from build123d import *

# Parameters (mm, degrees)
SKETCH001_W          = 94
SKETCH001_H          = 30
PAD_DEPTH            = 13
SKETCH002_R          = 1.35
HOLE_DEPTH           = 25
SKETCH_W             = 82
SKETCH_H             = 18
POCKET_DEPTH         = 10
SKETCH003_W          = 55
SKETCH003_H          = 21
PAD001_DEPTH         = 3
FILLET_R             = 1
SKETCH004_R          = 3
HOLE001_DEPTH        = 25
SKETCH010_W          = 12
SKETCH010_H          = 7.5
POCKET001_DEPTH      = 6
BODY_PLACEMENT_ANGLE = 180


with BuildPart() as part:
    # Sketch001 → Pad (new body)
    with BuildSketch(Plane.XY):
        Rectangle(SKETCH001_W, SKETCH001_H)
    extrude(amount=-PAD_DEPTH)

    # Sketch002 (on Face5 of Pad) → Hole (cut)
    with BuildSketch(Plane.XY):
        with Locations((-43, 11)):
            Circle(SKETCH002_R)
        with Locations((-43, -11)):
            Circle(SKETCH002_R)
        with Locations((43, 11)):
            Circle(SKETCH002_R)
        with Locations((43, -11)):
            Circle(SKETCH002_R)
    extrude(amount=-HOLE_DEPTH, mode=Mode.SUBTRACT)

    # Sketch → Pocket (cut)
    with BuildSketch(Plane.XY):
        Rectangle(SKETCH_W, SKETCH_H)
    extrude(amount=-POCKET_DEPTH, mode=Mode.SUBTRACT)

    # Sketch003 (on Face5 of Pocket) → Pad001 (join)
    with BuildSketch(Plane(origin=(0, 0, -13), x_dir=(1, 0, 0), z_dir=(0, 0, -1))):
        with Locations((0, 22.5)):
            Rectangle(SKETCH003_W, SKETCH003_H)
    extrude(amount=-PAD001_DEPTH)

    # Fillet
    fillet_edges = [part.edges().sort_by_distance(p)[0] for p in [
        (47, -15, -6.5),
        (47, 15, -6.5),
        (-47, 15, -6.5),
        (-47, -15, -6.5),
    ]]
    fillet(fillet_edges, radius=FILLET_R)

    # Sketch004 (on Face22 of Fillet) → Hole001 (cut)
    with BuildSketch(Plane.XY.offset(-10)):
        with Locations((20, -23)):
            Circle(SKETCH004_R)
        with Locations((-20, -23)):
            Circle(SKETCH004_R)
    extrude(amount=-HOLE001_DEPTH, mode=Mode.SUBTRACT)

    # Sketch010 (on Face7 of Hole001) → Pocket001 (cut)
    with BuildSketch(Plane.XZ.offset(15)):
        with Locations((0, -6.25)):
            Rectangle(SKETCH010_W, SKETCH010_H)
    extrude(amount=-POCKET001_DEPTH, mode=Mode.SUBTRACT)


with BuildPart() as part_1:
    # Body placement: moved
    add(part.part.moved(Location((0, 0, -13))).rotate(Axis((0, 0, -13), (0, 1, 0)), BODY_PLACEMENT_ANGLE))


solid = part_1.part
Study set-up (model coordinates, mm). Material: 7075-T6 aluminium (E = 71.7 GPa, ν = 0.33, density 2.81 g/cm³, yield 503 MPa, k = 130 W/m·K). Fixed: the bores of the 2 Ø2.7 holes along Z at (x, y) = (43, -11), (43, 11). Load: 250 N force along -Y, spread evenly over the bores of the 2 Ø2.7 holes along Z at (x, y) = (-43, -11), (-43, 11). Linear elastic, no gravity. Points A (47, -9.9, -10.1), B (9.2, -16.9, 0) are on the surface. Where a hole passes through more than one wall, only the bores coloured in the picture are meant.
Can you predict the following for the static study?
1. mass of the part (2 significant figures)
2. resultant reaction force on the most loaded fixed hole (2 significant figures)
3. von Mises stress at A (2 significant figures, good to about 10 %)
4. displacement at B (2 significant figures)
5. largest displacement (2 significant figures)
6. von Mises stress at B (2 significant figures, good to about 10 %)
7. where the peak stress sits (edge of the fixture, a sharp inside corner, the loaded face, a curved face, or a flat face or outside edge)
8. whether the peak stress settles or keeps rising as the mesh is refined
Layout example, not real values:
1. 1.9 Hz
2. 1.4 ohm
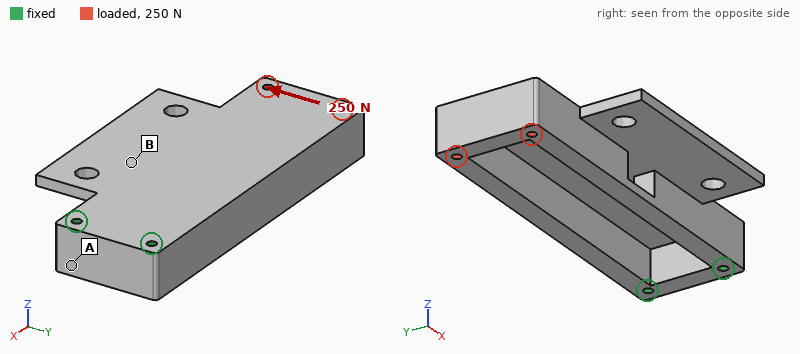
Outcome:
1. 67 g
2. 900 N
3. 3.1 MPa
4. 21 µm
5. 93 µm
6. 7.7 MPa
7. edge of the fixture
8. keeps rising
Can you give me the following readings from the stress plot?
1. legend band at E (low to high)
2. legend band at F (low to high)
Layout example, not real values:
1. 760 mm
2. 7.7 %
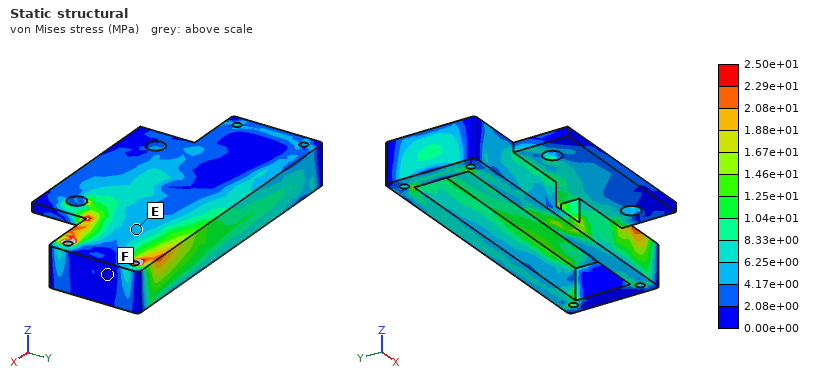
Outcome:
1. 4.17e+00 to 6.25e+00 MPa
2. 0.00e+00 to 2.08e+00 MPa
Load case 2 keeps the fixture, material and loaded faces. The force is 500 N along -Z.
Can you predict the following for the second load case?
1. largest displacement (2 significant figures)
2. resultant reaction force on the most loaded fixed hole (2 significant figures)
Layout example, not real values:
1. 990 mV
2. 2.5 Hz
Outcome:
1. 0.54 mm
2. 350 N
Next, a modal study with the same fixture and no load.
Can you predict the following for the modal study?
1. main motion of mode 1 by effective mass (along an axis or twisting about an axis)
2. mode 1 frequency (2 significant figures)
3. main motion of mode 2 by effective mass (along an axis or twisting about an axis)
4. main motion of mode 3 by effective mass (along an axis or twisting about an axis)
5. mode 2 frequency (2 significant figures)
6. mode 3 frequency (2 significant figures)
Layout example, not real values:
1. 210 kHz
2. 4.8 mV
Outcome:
1. along Z
2. 1100 Hz
3. along Y
4. along Y
5. 1800 Hz
6. 3200 Hz
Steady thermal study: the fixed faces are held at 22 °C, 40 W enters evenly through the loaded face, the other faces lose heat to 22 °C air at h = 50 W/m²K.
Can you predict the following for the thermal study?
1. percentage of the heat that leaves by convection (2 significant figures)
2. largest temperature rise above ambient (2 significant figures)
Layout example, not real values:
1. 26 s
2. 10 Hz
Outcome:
1. 53 %
2. 78 K
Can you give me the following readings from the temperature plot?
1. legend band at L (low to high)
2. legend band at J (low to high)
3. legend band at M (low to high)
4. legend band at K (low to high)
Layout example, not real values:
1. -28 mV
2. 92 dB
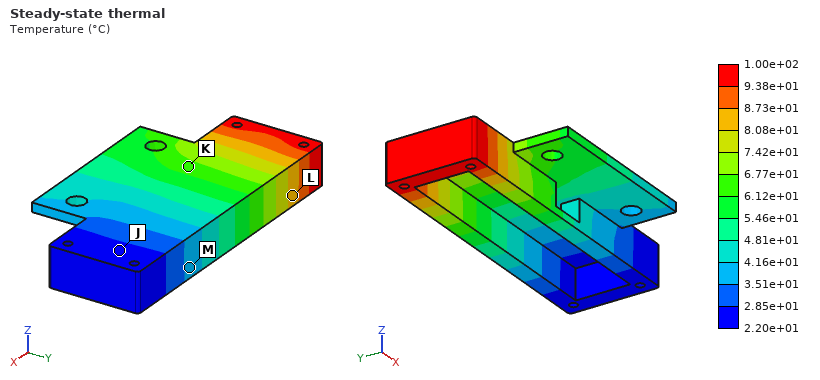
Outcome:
1. 8.08e+01 to 8.73e+01 °C
2. 2.20e+01 to 2.85e+01 °C
3. 3.51e+01 to 4.16e+01 °C
4. 6.12e+01 to 6.77e+01 °C
